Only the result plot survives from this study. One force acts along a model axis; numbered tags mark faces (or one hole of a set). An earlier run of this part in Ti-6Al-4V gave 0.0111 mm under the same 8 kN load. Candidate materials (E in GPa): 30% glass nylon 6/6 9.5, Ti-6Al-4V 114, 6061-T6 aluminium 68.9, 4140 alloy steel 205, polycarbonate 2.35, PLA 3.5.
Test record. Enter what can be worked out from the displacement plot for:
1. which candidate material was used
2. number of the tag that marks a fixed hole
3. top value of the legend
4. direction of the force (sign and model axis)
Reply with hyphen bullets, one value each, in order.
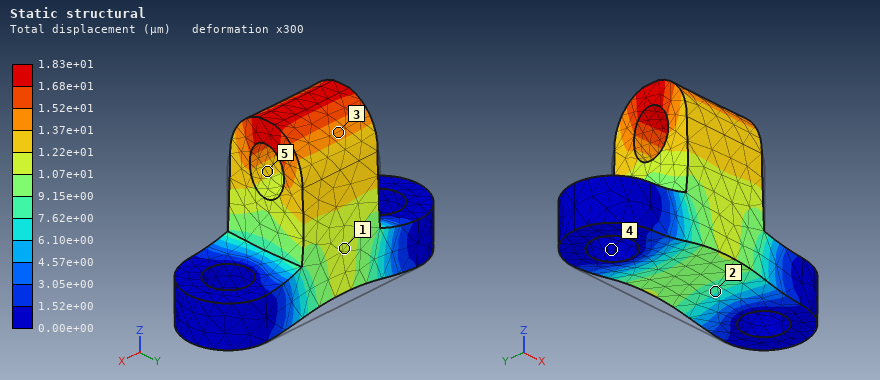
- 6061-T6 aluminium
- 4
- 1.83e+01 µm
- +Z
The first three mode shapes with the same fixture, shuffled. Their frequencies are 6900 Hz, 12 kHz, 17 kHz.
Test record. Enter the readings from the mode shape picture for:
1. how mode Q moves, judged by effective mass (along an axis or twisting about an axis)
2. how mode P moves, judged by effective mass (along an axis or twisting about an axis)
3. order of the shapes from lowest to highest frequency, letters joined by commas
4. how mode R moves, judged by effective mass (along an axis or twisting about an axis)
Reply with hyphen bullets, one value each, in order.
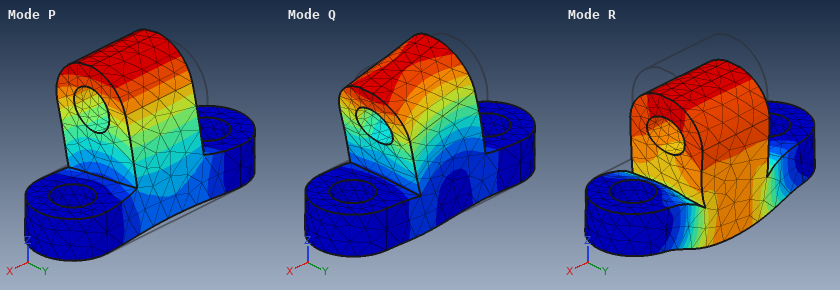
- along X
- along Y
- P, Q, R
- along Z
